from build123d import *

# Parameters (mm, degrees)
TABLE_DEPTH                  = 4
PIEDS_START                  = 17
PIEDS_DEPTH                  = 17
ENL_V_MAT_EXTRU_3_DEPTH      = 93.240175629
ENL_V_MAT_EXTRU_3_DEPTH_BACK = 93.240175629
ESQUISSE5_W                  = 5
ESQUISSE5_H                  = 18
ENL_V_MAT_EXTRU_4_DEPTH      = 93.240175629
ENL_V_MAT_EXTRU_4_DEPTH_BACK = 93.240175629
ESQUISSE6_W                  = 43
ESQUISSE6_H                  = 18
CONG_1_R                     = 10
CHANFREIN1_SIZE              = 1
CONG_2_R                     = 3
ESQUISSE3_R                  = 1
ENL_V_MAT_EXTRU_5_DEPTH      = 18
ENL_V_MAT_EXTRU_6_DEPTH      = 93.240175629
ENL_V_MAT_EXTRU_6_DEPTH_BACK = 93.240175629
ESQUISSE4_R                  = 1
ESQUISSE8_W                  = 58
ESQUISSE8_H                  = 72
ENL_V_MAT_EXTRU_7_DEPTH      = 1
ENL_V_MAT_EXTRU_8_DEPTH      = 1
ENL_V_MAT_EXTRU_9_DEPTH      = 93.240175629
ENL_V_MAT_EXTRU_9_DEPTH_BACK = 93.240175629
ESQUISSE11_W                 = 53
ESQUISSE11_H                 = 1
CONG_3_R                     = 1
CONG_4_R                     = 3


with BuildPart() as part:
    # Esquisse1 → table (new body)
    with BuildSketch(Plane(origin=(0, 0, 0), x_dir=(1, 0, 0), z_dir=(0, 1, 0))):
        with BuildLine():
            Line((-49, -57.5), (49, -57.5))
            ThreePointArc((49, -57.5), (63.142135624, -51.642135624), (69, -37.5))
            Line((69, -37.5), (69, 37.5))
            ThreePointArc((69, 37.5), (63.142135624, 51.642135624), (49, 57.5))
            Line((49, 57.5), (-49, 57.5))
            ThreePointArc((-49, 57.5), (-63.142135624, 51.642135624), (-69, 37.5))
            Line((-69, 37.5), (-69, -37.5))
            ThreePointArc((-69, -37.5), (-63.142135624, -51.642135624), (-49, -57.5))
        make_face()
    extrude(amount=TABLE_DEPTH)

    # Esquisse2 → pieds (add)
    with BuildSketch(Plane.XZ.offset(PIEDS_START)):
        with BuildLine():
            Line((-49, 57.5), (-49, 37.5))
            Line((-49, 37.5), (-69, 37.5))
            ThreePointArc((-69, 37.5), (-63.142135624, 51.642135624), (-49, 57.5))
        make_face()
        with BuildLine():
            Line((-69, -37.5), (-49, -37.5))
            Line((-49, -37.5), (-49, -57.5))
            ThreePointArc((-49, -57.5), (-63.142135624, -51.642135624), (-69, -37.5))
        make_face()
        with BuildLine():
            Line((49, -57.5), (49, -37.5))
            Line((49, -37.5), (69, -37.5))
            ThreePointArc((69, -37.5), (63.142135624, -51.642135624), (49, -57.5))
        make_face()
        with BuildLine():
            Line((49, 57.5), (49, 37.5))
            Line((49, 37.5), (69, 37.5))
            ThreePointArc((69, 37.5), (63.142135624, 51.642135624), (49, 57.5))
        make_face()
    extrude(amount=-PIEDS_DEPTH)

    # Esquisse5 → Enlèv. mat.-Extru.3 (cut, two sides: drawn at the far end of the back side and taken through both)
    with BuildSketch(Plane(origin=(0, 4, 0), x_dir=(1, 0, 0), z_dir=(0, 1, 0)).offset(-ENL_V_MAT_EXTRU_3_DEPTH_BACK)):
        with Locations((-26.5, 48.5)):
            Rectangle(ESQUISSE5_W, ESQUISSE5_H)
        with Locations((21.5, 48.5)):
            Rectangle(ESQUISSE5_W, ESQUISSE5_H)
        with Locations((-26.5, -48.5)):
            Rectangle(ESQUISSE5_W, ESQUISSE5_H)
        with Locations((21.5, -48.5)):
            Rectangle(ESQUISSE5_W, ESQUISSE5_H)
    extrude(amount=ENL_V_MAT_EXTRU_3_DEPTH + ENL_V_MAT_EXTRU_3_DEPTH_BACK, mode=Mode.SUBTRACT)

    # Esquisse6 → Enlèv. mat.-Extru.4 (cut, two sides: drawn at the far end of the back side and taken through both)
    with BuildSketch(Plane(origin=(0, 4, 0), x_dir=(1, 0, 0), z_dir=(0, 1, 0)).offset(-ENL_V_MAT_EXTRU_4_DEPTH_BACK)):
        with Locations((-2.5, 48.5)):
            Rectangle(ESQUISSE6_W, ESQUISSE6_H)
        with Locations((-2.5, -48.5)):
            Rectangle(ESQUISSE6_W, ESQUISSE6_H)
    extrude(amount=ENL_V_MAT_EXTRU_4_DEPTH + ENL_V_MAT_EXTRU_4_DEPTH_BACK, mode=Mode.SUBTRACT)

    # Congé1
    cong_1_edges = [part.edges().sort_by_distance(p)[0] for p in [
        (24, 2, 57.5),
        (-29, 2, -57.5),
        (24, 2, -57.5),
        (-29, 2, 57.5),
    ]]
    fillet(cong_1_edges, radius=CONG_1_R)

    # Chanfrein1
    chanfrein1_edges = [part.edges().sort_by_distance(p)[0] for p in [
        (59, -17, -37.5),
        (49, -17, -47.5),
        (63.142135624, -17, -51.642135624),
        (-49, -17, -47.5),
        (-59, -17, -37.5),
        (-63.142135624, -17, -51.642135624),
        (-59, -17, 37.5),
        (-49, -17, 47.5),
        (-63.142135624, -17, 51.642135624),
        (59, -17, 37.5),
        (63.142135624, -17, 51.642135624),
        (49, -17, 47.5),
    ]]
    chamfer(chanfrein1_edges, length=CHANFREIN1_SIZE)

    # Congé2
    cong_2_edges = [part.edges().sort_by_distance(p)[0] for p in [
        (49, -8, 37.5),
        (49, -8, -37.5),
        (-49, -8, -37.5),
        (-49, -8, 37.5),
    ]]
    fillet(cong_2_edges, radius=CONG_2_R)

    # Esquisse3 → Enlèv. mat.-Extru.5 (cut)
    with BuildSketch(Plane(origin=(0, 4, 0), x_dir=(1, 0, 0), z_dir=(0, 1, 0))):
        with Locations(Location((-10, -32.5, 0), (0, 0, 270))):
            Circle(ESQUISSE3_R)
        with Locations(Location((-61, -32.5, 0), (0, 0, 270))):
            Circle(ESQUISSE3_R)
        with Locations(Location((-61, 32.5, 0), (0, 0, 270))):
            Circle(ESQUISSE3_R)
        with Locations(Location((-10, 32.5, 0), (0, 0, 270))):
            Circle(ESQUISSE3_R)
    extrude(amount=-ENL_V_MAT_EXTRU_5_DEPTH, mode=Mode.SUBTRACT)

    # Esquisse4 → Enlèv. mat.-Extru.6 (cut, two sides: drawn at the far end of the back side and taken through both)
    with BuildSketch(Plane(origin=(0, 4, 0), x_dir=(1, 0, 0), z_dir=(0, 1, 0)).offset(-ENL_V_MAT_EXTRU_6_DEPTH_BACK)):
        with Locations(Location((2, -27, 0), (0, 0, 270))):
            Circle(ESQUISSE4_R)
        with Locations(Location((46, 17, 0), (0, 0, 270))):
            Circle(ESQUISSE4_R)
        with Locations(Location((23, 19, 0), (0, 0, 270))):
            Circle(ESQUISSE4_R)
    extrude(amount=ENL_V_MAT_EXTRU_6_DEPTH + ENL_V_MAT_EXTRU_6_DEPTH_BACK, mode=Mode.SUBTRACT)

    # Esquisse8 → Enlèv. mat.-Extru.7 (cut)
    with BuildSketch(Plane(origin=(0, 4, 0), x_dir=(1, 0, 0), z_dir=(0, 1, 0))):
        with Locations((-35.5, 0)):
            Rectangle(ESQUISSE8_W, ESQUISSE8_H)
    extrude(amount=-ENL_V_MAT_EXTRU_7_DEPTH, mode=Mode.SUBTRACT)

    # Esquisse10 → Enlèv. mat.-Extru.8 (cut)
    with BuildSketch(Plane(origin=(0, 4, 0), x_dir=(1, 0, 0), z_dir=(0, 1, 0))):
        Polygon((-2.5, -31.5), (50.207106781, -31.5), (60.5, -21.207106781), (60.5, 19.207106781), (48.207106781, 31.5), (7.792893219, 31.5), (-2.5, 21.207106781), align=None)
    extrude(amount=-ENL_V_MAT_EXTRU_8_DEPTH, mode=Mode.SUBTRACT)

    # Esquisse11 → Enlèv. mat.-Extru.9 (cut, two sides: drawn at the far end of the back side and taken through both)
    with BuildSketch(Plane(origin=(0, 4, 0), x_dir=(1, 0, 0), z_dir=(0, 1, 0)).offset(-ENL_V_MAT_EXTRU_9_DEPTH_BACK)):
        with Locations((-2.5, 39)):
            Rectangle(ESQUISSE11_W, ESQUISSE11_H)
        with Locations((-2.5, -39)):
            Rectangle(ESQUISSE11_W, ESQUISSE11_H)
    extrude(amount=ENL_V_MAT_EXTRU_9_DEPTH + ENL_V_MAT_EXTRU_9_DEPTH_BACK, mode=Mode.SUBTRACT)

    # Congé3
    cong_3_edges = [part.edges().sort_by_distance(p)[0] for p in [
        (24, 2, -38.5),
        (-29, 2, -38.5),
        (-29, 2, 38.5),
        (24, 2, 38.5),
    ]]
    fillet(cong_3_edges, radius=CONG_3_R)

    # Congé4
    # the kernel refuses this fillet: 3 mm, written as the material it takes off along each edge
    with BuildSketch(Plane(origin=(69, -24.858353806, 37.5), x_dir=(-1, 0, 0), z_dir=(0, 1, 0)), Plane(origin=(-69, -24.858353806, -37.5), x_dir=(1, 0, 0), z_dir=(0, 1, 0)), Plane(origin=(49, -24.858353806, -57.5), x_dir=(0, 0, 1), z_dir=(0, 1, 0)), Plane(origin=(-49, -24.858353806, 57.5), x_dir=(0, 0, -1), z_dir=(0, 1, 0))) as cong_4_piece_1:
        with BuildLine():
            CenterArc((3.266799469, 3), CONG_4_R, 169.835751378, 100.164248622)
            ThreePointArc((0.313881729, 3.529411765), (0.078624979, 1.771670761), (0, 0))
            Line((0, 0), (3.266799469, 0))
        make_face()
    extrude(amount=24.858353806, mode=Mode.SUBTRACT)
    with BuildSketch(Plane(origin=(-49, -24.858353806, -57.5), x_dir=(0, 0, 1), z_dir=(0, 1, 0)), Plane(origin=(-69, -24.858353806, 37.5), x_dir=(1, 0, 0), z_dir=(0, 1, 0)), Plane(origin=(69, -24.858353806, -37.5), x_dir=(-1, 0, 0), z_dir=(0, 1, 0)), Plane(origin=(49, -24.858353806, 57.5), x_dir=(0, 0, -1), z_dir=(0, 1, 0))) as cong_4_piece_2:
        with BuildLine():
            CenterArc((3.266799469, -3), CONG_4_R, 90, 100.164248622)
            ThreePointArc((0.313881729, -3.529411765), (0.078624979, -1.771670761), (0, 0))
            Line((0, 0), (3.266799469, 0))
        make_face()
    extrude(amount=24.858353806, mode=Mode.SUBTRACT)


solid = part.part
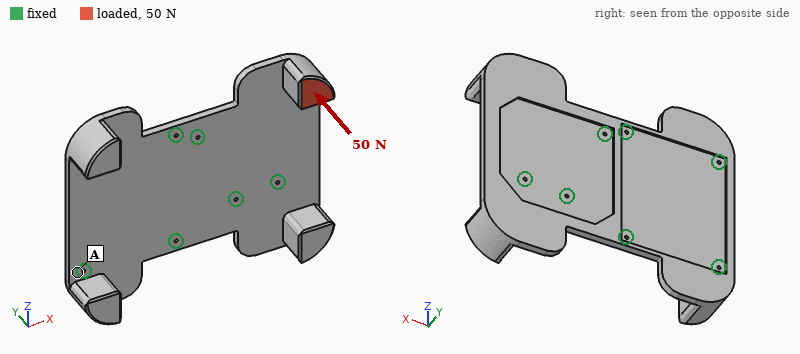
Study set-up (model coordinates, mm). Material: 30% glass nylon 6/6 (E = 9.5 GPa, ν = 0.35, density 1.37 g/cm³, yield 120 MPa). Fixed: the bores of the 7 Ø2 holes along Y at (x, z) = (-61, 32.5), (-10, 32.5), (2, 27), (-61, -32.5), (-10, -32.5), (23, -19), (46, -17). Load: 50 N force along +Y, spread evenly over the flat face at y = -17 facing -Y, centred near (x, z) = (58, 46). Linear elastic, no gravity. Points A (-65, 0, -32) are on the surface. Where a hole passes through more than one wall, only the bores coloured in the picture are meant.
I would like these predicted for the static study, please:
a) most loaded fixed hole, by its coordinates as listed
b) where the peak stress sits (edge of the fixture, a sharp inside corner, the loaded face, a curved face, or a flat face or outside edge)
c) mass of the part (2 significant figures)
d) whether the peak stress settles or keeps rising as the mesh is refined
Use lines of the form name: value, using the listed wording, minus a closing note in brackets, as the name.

most loaded fixed hole, by its coordinates as listed: (2, 27)
where the peak stress sits: edge of the fixture
mass of the part: 91 g
whether the peak stress settles or keeps rising as the mesh is refined: keeps rising
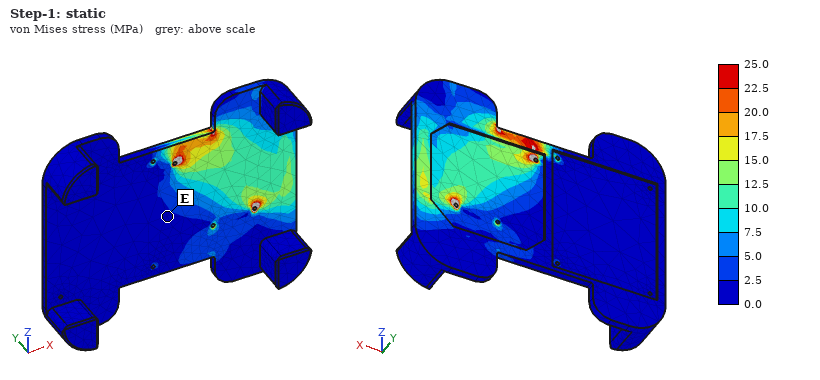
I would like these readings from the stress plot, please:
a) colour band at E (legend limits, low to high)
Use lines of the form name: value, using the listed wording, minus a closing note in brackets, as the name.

colour band at E: 0.0 to 2.5 MPa
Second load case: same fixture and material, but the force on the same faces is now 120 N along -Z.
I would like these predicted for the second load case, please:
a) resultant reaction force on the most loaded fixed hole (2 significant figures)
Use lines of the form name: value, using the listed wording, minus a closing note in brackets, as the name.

resultant reaction force on the most loaded fixed hole: 75 N
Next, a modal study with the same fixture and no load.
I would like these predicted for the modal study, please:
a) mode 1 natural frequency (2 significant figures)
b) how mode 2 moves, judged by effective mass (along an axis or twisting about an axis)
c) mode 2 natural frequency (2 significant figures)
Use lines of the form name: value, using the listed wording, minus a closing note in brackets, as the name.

mode 1 natural frequency: 250 Hz
how mode 2 moves, judged by effective mass: along Y
mode 2 natural frequency: 470 Hz
